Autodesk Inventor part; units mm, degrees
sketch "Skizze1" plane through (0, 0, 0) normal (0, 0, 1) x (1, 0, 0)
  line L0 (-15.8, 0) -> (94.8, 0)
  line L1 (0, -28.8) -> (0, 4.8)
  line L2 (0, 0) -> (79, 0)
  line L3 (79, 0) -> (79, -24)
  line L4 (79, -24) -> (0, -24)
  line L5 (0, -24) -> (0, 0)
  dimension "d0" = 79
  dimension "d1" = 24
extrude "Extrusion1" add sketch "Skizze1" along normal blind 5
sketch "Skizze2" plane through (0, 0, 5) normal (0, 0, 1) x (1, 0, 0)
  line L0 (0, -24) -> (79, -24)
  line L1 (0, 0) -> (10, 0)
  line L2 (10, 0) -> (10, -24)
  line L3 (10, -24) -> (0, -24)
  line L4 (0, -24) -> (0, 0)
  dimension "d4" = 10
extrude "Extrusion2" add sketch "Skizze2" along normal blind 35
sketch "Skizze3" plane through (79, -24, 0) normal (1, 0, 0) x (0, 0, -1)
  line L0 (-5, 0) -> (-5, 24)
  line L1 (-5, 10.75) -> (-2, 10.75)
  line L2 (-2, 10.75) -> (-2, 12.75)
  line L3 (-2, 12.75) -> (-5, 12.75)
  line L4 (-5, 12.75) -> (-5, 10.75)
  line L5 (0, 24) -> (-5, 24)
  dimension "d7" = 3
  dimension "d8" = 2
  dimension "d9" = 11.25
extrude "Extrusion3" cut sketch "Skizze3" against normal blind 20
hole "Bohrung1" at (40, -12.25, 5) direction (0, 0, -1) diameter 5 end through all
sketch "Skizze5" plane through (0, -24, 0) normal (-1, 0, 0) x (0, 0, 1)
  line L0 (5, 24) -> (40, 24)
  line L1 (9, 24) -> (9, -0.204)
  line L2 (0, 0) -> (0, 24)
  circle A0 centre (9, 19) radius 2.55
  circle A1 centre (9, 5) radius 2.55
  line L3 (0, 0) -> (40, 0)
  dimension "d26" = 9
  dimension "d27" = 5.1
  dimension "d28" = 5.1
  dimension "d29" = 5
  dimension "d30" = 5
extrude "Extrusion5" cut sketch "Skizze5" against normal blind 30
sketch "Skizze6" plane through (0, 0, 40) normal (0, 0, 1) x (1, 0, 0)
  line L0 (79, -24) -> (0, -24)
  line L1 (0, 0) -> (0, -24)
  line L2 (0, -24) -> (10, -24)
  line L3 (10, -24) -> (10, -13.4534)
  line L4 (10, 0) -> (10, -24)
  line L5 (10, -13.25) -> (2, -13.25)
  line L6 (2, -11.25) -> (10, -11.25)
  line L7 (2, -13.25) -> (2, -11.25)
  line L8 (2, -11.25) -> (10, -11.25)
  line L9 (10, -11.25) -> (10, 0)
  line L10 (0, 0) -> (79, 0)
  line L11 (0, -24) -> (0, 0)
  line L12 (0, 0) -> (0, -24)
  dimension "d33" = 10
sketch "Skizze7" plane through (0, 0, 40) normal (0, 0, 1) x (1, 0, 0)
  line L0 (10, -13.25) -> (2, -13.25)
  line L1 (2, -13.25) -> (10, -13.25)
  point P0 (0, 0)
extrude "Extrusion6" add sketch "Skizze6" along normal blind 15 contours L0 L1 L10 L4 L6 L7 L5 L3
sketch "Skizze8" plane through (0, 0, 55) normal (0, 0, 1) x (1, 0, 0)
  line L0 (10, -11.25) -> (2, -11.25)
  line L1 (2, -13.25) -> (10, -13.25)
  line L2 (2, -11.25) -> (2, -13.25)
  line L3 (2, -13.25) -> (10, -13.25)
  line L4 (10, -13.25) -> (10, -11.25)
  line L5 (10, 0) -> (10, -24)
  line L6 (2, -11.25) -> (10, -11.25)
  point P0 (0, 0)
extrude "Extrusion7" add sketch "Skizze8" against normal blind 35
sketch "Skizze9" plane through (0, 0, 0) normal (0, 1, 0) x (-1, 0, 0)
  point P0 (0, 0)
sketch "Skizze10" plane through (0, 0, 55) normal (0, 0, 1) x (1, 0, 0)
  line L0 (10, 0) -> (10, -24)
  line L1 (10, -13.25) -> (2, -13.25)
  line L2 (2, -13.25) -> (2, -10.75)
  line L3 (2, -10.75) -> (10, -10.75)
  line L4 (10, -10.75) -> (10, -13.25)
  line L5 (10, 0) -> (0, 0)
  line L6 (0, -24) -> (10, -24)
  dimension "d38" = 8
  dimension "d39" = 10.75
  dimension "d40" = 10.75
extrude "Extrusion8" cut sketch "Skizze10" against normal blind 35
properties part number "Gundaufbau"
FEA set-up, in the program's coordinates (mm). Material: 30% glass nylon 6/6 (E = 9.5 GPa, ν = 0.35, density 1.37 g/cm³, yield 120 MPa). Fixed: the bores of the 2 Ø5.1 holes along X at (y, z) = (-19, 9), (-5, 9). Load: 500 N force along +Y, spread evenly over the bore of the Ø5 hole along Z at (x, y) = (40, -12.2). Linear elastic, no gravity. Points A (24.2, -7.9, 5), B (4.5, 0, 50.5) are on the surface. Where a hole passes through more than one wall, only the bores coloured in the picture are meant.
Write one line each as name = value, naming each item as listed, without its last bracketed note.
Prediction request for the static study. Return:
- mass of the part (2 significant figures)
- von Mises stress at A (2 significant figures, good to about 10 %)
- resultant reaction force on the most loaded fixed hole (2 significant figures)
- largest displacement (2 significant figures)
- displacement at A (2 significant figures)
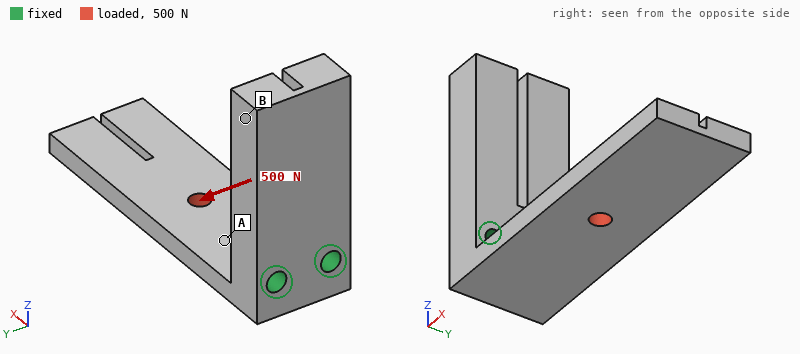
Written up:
mass of the part = 28 g
von Mises stress at A = 12 MPa
resultant reaction force on the most loaded fixed hole = 940 N
largest displacement = 0.50 mm
displacement at A = 0.10 mm
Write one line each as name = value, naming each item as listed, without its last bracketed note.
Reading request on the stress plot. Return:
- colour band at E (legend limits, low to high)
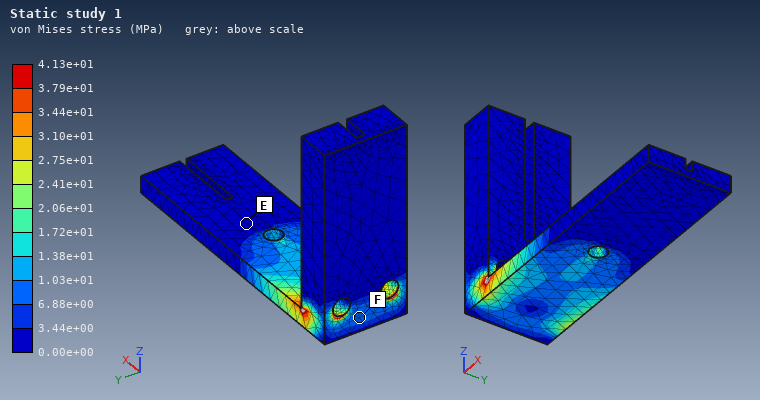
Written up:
colour band at E = 0.00e+00 to 3.44e+00 MPa
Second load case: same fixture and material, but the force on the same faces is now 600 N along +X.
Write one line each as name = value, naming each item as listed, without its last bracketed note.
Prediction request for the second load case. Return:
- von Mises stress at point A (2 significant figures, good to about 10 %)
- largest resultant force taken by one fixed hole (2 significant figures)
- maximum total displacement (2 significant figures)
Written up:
von Mises stress at point A = 5.2 MPa
largest resultant force taken by one fixed hole = 310 N
maximum total displacement = 85 µm
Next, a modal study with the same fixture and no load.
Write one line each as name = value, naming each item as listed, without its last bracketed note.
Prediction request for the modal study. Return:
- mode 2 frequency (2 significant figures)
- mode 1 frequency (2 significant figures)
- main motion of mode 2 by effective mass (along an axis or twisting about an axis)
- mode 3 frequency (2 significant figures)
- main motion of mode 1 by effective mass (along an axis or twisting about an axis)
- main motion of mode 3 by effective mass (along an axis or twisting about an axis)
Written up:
mode 2 frequency = 1600 Hz
mode 1 frequency = 420 Hz
main motion of mode 2 by effective mass = along Y
mode 3 frequency = 2100 Hz
main motion of mode 1 by effective mass = along Z
main motion of mode 3 by effective mass = along X
